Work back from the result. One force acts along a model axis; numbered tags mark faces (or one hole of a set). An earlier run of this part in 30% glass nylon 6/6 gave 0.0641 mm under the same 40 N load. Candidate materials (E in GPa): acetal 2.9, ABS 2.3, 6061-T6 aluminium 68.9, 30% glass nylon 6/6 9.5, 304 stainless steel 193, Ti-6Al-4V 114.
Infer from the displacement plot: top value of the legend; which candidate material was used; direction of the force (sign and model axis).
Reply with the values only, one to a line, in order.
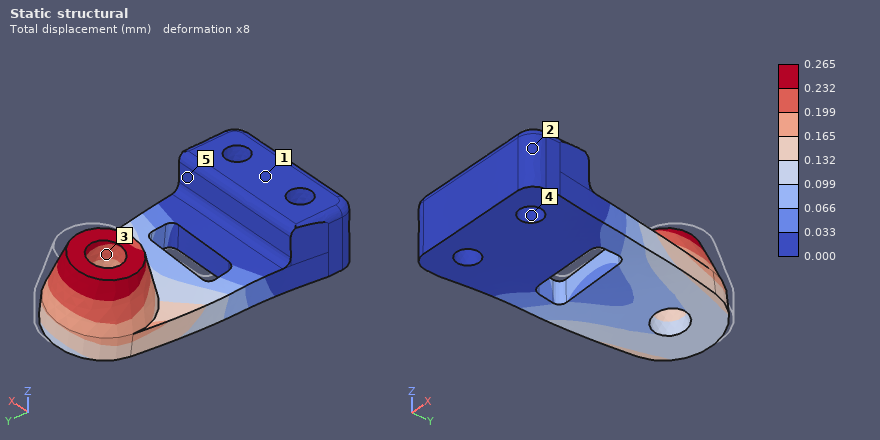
0.265 mm
ABS
-X
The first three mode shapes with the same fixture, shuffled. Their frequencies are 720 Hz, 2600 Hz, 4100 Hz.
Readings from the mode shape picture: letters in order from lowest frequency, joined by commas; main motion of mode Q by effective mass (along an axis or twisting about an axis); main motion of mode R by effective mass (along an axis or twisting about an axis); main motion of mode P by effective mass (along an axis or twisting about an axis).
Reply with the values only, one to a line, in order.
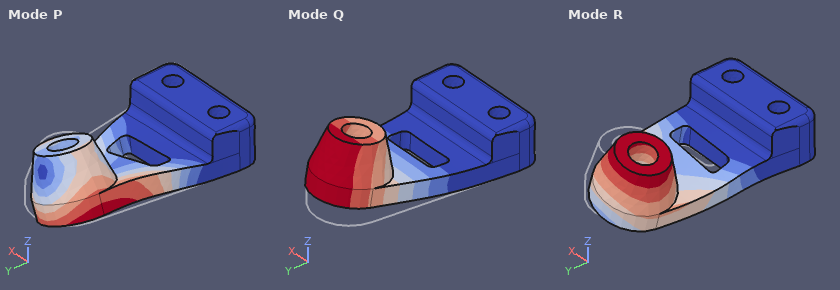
Q, R, P
along Z
along X
along X
